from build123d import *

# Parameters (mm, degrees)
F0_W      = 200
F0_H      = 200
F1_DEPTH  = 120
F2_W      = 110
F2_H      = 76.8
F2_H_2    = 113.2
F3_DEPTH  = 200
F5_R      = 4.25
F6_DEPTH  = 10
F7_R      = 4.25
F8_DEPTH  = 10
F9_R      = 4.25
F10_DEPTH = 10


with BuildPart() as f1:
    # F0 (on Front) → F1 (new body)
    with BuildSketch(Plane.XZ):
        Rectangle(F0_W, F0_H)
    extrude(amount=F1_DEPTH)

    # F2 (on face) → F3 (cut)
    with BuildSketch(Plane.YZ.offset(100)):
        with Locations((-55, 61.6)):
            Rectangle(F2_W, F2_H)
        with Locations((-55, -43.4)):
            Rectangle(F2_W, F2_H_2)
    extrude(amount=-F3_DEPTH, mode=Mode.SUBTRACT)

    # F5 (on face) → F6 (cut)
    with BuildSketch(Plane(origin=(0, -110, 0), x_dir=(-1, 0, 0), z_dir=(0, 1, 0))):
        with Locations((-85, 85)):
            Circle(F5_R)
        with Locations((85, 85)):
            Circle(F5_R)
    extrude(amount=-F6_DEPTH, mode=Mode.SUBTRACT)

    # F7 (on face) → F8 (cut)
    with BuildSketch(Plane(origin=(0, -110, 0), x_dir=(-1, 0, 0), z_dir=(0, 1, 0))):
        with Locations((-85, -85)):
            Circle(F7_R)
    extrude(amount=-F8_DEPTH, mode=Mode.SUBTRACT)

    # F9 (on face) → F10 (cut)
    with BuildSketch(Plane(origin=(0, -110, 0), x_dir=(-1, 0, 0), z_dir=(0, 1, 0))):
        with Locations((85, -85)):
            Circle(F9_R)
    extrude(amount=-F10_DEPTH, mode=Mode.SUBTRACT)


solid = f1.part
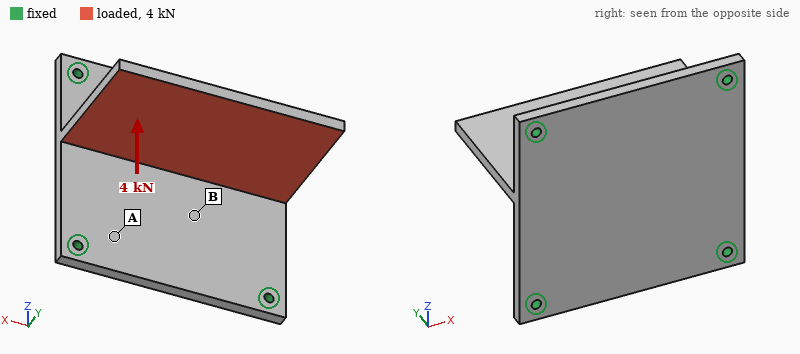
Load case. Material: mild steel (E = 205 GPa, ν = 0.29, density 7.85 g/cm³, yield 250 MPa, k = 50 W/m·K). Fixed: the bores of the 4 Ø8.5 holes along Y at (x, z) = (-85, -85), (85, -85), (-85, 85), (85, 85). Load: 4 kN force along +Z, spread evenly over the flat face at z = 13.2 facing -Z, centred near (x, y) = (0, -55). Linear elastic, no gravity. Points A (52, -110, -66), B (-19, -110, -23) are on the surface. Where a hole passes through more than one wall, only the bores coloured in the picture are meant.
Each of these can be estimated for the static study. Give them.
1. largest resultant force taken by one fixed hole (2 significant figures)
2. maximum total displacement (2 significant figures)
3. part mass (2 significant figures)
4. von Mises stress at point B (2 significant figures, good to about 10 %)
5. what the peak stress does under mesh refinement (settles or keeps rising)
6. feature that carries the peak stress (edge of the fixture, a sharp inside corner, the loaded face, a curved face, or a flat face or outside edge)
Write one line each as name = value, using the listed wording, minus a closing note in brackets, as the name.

largest resultant force taken by one fixed hole = 1.4 kN
maximum total displacement = 0.30 mm
part mass = 4.8 kg
von Mises stress at point B = 17 MPa
what the peak stress does under mesh refinement = keeps rising
feature that carries the peak stress = edge of the fixture
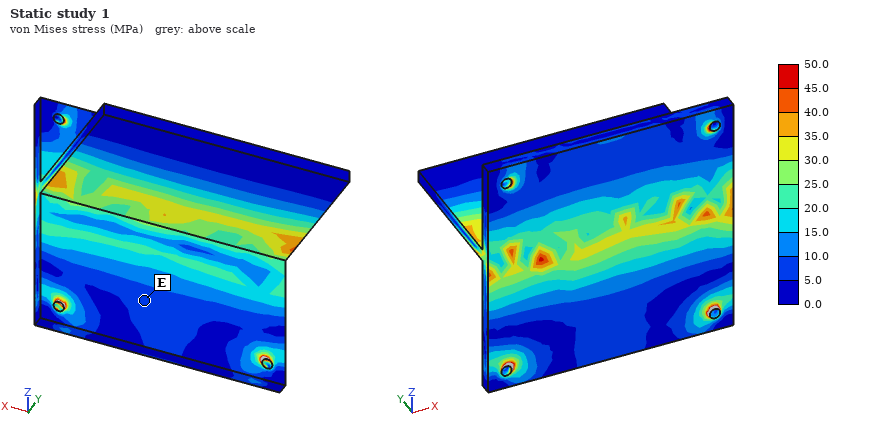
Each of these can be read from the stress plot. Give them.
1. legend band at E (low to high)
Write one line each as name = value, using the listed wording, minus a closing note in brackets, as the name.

legend band at E = 5.0 to 10.0 MPa
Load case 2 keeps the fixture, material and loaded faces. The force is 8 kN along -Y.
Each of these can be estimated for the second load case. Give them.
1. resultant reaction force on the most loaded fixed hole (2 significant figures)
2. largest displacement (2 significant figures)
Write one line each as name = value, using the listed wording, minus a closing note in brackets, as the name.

resultant reaction force on the most loaded fixed hole = 2.4 kN
largest displacement = 0.15 mm
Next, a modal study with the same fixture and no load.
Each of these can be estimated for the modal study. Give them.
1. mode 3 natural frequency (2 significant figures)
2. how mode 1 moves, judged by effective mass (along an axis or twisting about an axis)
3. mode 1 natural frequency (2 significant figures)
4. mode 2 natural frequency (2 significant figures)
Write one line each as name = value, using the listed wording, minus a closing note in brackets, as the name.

mode 3 natural frequency = 920 Hz
how mode 1 moves, judged by effective mass = along Z
mode 1 natural frequency = 540 Hz
mode 2 natural frequency = 900 Hz
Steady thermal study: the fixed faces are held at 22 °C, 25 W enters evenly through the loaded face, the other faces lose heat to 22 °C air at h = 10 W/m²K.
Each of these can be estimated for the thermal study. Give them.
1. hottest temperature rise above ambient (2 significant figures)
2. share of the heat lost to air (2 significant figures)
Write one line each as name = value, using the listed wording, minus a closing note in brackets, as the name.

hottest temperature rise above ambient = 21 K
share of the heat lost to air = 39 %
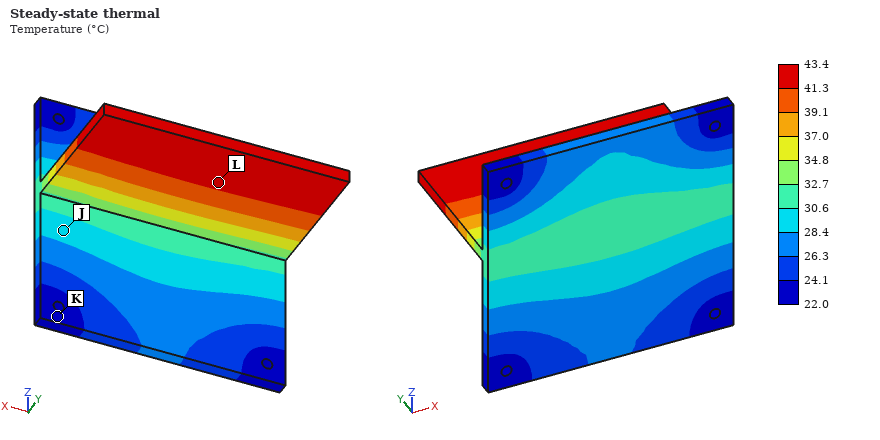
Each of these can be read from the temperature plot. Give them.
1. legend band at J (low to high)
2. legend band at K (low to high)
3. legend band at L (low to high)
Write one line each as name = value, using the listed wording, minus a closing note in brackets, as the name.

legend band at J = 28.4 to 30.6 °C
legend band at K = 22.0 to 24.1 °C
legend band at L = 41.3 to 43.4 °C
